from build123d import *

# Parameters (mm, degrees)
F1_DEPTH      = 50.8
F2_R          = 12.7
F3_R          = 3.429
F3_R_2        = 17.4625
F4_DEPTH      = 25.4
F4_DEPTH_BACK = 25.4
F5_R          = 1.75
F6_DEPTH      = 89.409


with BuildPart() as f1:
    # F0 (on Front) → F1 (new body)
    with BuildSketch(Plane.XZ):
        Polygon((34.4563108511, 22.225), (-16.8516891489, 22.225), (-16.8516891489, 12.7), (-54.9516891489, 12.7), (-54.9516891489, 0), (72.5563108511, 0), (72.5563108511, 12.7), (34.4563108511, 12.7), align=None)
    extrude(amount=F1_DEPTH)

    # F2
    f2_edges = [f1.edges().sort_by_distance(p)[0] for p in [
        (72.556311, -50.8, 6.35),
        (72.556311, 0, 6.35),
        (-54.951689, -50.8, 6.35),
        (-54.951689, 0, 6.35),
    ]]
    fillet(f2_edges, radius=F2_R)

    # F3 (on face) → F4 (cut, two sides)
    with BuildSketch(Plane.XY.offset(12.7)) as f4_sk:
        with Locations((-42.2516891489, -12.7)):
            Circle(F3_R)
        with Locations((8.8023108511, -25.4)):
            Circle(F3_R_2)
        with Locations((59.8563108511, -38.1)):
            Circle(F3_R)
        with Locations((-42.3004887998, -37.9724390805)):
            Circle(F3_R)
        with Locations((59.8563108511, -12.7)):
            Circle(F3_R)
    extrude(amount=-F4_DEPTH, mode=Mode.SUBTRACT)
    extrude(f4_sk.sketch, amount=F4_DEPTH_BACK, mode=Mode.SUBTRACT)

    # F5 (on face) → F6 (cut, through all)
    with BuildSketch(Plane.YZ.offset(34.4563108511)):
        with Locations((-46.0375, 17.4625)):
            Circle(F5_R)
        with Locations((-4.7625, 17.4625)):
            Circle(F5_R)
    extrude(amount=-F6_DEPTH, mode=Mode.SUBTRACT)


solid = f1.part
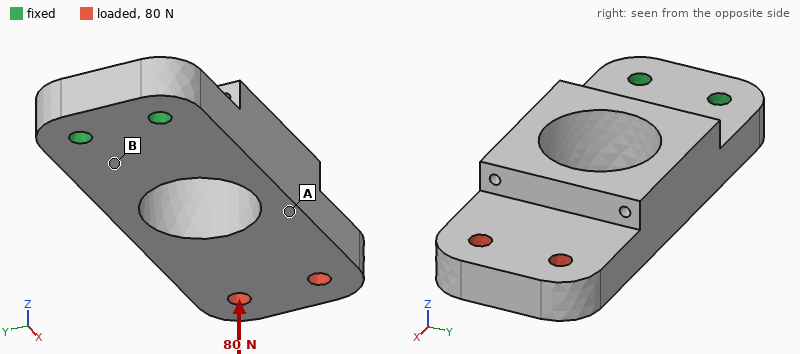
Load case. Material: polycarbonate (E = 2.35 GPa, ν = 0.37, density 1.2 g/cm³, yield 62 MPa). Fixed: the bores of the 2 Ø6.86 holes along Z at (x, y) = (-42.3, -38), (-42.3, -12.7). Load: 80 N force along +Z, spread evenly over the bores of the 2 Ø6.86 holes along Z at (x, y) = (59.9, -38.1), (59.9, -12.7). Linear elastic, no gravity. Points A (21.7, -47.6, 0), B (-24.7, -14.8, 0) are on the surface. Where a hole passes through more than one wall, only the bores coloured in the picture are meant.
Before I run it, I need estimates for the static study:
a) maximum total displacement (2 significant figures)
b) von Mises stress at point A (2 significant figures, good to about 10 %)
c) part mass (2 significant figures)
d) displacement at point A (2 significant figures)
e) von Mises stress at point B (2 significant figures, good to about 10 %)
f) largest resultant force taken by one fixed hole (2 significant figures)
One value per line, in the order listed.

1.4 mm
1.9 MPa
97 g
0.60 mm
4.6 MPa
41 N
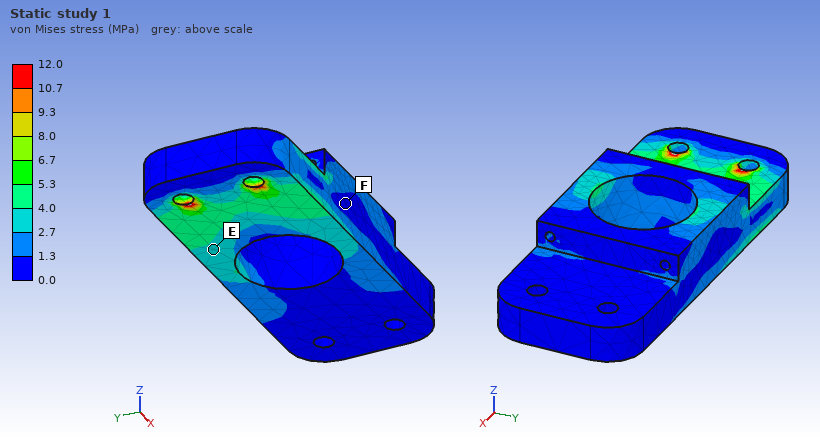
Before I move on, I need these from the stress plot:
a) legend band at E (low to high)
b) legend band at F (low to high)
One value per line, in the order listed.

2.7 to 4.0 MPa
0.0 to 1.3 MPa
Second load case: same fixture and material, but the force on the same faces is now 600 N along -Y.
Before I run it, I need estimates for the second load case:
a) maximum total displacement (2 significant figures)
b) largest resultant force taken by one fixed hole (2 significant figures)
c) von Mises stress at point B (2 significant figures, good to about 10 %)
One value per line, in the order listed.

1.4 mm
2.1 kN
4.3 MPa
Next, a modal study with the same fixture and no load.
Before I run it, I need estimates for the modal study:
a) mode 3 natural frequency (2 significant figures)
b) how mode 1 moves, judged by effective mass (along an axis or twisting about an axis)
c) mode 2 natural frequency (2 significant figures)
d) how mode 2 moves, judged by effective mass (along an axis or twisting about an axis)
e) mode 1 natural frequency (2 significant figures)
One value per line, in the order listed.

890 Hz
along Z
590 Hz
along Y
230 Hz
